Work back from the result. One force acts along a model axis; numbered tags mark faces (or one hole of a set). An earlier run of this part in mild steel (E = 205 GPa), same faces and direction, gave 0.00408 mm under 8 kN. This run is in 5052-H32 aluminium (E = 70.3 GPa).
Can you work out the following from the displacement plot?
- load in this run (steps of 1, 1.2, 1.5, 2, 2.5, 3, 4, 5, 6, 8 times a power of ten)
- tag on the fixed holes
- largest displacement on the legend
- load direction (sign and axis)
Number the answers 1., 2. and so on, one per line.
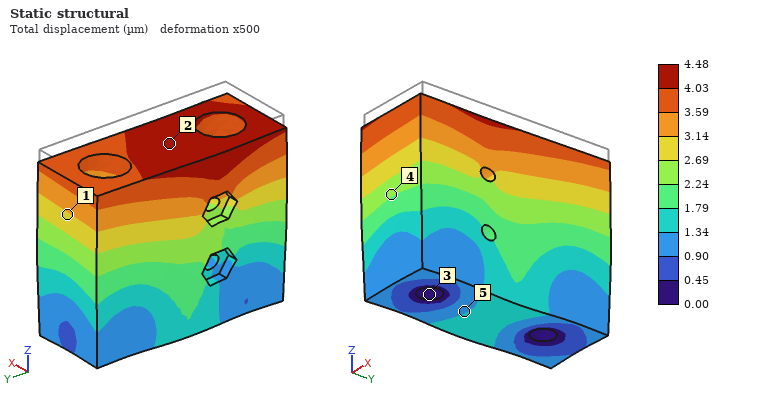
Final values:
1. 3 kN
2. 3
3. 4.48 µm
4. -Z
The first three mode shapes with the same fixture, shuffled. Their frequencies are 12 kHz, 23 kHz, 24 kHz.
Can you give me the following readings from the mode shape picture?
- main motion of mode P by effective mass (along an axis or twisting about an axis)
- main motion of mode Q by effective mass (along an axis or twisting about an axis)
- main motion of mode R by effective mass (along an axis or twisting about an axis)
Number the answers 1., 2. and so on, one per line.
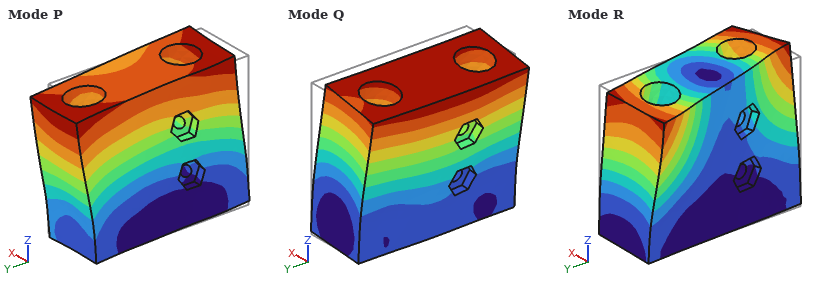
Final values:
1. along Y
2. along X
3. twisting about Z
